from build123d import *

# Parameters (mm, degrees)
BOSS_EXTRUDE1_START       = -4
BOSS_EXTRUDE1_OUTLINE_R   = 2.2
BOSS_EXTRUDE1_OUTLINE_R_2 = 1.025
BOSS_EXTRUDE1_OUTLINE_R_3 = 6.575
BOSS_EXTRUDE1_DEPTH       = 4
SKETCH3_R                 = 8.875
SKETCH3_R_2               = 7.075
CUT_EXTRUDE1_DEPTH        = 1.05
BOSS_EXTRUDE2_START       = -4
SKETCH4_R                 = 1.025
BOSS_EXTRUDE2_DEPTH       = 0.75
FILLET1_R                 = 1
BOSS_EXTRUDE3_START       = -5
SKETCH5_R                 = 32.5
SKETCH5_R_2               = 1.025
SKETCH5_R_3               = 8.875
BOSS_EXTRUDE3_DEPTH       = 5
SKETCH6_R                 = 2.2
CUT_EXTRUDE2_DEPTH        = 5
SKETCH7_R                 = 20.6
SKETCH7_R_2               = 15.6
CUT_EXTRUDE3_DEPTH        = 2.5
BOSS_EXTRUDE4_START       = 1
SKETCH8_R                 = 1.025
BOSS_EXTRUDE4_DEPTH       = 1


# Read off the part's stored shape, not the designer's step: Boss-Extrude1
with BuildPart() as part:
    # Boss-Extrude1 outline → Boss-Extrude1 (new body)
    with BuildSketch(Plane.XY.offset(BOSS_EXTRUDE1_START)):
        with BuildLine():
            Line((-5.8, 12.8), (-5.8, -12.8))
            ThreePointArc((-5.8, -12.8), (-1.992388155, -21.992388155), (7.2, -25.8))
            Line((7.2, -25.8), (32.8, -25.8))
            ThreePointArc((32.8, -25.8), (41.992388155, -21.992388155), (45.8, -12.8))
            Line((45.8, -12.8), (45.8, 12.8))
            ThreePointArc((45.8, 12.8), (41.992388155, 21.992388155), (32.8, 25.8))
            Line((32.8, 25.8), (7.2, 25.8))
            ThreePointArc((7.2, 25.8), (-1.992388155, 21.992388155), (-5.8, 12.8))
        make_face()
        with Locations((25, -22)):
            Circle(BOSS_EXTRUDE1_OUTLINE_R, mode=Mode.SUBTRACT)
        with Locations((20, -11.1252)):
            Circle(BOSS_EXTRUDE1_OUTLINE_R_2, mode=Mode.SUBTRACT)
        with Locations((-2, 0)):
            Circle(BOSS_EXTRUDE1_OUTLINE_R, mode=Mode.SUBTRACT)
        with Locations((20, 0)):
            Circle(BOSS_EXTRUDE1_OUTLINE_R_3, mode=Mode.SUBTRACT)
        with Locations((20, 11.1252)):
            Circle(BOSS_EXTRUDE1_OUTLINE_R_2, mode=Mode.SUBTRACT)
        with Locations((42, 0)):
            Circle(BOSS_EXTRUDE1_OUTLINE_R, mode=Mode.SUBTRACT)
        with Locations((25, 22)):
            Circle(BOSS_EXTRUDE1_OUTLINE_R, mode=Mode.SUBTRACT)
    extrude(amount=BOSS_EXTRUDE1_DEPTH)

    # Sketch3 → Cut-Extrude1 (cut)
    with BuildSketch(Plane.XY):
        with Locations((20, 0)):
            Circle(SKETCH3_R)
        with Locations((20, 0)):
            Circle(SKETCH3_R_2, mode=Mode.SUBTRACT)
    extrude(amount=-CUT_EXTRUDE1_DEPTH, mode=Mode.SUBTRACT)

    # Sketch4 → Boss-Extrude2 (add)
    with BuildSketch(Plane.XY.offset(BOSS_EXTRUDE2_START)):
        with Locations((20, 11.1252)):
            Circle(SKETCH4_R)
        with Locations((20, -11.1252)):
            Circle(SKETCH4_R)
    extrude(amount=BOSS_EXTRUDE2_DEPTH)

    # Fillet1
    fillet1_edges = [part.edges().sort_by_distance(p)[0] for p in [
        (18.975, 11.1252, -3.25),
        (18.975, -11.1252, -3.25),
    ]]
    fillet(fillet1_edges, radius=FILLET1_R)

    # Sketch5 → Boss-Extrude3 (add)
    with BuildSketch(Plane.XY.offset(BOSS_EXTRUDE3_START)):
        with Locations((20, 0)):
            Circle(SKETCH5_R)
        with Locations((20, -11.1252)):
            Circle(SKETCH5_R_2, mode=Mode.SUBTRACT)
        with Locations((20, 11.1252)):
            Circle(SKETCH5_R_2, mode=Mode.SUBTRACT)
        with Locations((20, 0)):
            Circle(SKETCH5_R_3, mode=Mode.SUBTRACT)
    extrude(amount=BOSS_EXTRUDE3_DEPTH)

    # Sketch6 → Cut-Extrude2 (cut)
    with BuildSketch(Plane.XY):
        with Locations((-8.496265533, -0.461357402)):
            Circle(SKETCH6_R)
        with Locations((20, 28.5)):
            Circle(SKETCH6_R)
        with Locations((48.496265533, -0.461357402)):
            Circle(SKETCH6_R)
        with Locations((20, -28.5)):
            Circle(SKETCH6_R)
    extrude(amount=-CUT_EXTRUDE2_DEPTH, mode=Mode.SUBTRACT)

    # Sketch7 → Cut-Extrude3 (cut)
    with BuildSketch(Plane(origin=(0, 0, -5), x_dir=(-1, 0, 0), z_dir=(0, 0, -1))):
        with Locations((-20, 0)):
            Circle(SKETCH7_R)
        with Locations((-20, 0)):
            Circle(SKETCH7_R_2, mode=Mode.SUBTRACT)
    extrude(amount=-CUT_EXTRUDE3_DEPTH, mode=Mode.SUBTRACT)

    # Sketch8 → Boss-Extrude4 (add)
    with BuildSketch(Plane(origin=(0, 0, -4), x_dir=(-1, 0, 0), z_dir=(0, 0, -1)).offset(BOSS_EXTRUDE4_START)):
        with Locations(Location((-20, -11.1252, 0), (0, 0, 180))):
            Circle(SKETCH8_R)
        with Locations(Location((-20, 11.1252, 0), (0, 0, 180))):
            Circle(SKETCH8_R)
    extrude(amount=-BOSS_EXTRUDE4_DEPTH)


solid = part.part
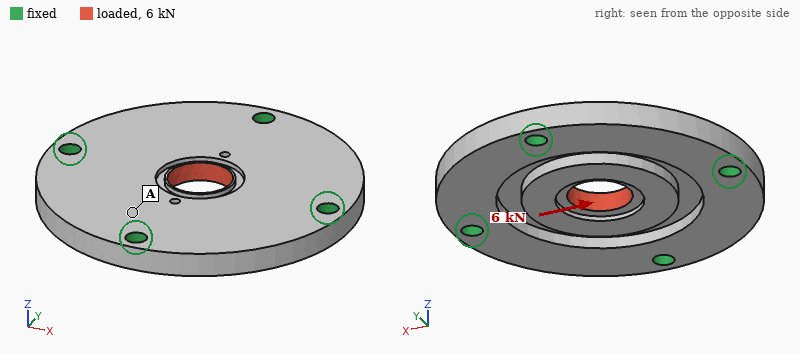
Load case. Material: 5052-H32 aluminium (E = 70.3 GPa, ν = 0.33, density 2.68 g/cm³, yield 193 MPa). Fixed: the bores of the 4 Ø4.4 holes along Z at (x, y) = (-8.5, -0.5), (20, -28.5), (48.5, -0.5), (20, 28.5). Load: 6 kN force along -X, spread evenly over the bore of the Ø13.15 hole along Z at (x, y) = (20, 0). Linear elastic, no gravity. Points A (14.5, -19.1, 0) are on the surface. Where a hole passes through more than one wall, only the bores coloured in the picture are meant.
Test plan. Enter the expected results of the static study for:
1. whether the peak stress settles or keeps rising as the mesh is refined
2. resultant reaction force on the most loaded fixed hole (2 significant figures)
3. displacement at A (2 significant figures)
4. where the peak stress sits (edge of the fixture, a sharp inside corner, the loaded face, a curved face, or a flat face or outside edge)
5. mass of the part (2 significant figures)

keeps rising
1.8 kN
4.8 µm
a sharp inside corner
37 g
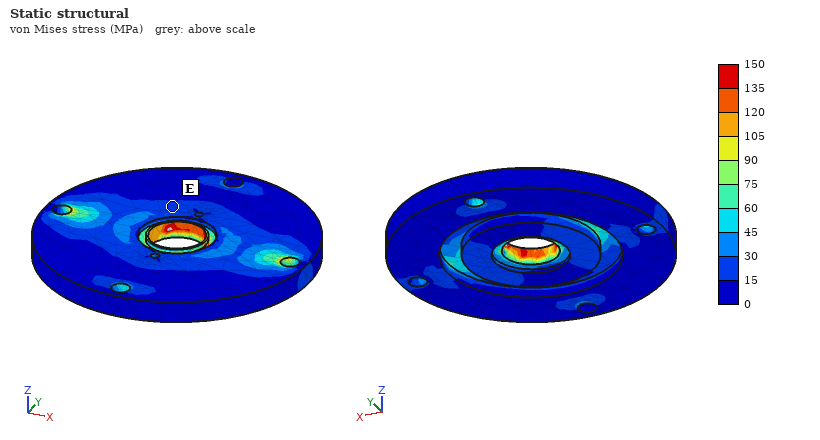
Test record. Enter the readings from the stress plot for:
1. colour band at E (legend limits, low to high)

15 to 30 MPa
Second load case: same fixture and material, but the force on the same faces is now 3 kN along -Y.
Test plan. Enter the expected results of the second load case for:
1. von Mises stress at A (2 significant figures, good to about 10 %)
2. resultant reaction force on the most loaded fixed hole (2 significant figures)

14 MPa
900 N
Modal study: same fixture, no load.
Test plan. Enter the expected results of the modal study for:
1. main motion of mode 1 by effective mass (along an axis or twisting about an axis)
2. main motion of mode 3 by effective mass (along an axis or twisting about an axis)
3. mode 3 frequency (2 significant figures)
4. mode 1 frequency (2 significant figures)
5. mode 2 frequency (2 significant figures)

along Z
twisting about X
13 kHz
11 kHz
13 kHz
